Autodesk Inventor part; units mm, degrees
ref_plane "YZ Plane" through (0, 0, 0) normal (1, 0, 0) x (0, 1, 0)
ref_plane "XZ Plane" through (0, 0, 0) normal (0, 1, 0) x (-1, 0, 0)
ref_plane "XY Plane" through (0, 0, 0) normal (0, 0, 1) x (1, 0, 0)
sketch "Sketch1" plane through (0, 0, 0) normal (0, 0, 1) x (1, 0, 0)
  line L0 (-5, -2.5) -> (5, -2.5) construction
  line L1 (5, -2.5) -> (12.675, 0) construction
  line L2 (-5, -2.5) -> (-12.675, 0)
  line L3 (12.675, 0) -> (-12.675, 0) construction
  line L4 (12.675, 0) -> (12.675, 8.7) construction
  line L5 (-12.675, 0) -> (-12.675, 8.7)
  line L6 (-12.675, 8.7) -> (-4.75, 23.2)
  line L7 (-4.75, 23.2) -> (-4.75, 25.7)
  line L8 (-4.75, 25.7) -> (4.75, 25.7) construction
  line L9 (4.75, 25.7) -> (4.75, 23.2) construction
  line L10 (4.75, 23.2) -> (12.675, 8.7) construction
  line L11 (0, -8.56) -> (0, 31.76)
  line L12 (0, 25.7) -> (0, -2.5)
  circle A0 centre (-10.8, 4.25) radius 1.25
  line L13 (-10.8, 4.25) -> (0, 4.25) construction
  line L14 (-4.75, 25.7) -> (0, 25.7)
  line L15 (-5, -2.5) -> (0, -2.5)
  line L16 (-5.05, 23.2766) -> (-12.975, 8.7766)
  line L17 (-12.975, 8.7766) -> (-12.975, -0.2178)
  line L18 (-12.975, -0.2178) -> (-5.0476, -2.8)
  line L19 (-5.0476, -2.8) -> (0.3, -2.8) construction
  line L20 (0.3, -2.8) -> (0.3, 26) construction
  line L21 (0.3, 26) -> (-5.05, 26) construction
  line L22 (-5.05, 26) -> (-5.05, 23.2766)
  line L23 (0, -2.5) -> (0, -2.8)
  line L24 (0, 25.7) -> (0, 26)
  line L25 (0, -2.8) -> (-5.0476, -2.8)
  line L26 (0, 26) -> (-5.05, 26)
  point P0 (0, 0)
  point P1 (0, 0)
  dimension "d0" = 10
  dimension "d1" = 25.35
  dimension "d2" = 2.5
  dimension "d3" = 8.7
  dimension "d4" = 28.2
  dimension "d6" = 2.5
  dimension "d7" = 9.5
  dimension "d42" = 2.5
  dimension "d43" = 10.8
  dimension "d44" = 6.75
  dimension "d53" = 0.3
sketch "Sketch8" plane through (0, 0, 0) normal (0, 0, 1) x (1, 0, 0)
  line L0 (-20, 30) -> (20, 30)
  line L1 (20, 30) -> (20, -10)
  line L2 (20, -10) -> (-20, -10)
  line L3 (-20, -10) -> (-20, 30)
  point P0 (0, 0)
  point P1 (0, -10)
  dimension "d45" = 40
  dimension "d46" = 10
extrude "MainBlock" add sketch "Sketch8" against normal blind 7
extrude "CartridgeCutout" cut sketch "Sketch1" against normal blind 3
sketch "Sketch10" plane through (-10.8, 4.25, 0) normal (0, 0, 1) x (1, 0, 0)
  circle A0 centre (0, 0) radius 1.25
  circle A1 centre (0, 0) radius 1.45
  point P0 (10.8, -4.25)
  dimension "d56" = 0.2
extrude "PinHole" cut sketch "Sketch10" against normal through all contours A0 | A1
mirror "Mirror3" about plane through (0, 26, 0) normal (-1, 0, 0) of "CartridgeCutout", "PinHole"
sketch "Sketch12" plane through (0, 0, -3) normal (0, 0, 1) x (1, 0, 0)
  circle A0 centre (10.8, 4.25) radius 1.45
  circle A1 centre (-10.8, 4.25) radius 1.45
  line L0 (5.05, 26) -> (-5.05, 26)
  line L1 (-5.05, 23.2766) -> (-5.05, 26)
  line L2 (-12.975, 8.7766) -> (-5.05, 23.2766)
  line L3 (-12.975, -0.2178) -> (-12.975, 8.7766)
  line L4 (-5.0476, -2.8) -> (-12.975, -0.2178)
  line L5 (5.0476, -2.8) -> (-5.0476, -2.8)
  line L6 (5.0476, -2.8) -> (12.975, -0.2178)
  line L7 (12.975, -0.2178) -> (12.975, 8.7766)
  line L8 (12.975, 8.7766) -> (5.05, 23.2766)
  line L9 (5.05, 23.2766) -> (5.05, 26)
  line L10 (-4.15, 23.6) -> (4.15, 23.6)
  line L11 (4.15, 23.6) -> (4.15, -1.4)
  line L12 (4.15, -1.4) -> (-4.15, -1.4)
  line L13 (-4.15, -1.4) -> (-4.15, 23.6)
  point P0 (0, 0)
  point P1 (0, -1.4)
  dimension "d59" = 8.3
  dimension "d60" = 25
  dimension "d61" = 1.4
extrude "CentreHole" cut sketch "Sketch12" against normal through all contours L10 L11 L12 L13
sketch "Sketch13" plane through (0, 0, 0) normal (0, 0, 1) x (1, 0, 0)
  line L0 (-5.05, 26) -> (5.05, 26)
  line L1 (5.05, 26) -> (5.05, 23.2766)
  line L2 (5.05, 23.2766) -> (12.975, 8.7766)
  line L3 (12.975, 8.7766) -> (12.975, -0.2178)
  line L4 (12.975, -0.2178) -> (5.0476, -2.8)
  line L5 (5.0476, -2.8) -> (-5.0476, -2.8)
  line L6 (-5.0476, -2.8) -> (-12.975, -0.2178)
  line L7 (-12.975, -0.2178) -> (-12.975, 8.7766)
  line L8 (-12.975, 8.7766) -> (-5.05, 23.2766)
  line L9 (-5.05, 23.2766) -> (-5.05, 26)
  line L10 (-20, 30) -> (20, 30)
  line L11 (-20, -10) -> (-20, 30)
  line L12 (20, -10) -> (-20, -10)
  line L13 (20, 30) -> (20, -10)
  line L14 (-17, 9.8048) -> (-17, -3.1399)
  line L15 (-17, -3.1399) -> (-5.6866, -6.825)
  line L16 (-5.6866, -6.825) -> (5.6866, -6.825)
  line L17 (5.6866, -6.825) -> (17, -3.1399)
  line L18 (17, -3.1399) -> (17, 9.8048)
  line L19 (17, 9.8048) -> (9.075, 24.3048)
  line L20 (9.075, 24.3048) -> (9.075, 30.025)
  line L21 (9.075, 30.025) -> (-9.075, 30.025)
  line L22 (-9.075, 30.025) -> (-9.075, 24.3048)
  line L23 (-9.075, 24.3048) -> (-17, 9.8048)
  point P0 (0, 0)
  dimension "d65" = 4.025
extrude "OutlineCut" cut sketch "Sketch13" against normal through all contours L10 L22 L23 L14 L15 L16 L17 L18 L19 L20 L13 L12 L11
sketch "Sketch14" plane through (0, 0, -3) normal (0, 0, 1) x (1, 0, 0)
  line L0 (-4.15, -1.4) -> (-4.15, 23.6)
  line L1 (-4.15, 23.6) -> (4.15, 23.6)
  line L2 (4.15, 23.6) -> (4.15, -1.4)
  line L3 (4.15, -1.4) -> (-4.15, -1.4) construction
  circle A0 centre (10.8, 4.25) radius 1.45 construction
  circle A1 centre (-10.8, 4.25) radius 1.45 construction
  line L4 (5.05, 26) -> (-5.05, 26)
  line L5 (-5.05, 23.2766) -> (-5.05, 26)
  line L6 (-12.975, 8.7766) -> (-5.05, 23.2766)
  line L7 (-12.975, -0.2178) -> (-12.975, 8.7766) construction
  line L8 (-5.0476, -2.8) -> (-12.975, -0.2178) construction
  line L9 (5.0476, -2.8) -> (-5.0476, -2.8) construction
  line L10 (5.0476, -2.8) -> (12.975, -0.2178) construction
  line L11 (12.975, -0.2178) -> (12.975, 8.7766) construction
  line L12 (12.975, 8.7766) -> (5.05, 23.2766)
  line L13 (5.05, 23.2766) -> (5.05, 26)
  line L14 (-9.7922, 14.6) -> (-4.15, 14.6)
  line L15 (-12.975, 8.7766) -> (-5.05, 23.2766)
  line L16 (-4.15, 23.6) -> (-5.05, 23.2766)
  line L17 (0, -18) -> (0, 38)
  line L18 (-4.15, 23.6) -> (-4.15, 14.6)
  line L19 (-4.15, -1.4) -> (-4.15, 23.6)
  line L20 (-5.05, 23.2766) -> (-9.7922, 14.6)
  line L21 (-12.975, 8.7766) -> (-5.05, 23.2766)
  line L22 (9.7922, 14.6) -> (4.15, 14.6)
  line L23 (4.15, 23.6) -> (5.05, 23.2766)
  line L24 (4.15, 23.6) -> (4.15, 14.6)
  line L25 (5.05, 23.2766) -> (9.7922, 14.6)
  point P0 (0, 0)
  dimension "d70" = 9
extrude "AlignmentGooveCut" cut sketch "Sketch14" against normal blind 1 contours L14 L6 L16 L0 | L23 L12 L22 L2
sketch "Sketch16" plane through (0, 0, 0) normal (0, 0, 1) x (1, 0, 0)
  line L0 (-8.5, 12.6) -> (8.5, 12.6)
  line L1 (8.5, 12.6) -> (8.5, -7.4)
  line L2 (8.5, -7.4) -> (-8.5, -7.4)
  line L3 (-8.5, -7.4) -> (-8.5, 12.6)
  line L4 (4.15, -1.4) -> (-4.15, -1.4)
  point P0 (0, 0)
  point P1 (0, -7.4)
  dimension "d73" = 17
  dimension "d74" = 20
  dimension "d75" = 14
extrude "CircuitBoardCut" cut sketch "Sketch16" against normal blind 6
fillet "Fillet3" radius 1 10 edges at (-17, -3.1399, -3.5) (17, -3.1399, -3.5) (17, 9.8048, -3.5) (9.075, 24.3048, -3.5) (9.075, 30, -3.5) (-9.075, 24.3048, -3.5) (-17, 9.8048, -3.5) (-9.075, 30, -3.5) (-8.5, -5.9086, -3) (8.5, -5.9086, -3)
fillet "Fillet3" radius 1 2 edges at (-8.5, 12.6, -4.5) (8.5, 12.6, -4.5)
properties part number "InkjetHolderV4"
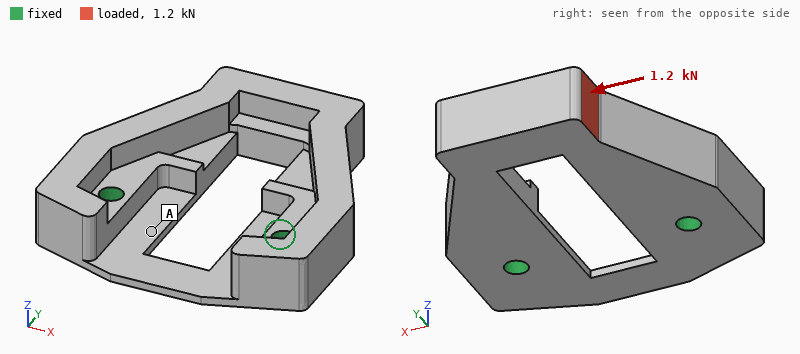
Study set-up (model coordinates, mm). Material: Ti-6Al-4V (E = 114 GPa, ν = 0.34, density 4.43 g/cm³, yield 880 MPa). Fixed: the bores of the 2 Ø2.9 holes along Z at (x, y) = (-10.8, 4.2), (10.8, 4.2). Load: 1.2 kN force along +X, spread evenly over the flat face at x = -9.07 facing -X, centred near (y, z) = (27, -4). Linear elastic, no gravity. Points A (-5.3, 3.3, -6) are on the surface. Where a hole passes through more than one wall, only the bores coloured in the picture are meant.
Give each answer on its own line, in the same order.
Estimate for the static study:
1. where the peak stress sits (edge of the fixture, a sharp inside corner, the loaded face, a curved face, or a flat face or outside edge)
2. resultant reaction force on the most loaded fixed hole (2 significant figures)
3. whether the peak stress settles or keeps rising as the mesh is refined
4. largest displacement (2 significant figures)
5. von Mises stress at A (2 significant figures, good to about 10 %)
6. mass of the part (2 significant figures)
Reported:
edge of the fixture
960 N
keeps rising
48 µm
36 MPa
16 g
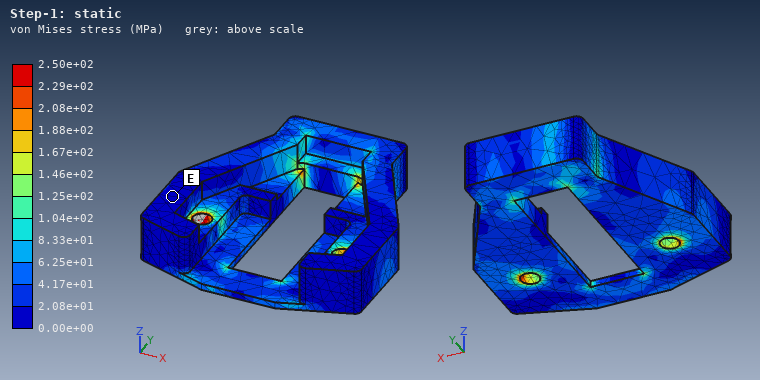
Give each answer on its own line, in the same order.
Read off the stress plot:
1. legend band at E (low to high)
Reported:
0.00e+00 to 2.08e+01 MPa
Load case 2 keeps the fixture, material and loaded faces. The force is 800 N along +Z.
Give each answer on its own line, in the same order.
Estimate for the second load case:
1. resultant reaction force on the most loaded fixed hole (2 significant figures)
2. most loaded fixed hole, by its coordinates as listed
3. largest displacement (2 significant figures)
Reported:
720 N
(-10.8, 4.2)
0.21 mm
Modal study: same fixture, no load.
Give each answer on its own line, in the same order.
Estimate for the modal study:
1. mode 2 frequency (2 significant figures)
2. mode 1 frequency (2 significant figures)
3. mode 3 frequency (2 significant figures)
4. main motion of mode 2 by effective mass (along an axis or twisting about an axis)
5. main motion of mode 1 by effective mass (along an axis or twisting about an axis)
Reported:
11 kHz
5500 Hz
14 kHz
along X
along Z
